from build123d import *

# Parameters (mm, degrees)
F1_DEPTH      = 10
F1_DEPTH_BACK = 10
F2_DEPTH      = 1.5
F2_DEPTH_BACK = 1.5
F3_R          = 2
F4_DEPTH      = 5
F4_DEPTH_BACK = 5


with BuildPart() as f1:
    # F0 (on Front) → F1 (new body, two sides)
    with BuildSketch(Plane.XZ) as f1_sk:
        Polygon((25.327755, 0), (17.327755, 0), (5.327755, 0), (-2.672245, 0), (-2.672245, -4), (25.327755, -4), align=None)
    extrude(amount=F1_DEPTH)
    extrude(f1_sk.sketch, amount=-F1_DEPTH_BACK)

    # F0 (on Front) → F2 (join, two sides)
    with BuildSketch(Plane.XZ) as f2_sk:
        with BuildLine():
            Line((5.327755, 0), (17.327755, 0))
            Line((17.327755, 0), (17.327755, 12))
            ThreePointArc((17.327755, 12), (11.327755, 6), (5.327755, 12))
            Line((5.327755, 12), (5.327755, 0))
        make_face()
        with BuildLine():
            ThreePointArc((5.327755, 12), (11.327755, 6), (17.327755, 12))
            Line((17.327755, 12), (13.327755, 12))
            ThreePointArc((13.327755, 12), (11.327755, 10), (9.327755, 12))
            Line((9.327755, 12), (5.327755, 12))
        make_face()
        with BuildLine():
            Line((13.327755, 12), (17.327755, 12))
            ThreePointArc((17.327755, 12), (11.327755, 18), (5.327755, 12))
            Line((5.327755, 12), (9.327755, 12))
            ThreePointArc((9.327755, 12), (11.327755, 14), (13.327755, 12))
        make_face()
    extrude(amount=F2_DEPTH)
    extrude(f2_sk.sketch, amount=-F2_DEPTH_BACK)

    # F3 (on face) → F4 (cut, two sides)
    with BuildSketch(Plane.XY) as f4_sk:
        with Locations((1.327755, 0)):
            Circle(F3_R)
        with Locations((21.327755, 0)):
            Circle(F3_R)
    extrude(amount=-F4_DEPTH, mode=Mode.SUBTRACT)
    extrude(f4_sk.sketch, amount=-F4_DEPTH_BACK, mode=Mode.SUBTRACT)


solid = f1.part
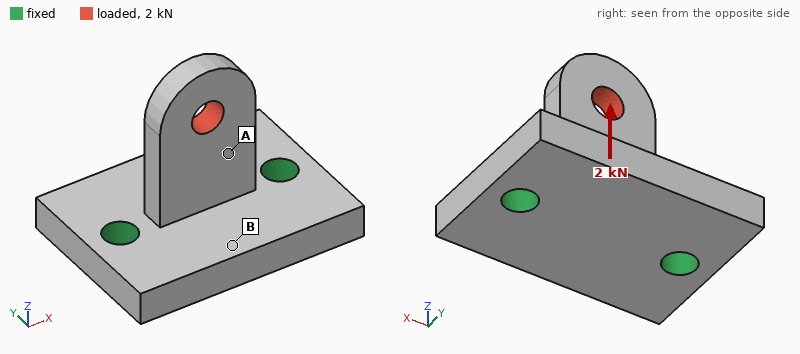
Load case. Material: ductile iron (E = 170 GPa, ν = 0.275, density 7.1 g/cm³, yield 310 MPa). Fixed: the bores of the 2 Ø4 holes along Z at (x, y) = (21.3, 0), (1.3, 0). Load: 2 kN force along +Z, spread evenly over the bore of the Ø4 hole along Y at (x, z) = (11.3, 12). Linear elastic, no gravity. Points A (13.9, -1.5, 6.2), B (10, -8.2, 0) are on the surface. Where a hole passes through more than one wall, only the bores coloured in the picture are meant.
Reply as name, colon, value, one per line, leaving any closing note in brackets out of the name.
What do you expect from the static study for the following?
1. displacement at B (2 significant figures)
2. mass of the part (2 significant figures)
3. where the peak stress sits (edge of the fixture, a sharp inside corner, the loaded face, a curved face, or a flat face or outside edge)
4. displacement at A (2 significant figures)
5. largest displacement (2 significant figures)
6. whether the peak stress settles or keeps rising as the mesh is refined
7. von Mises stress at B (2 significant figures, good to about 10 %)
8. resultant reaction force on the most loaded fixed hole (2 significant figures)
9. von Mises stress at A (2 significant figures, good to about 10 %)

displacement at B: 3.1 µm
mass of the part: 19 g
where the peak stress sits: edge of the fixture
displacement at A: 5.7 µm
largest displacement: 10.0 µm
whether the peak stress settles or keeps rising as the mesh is refined: keeps rising
von Mises stress at B: 22 MPa
resultant reaction force on the most loaded fixed hole: 1.0 kN
von Mises stress at A: 57 MPa
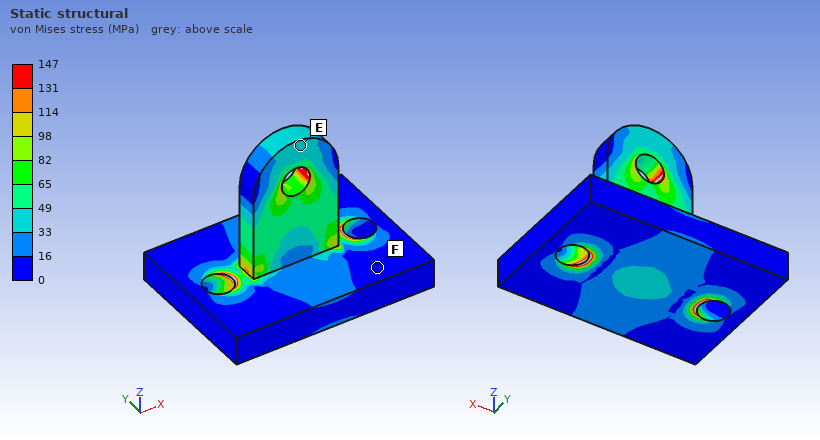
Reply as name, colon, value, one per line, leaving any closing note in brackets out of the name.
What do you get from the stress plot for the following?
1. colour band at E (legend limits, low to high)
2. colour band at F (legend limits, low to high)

colour band at E: 33 to 49 MPa
colour band at F: 0 to 16 MPa
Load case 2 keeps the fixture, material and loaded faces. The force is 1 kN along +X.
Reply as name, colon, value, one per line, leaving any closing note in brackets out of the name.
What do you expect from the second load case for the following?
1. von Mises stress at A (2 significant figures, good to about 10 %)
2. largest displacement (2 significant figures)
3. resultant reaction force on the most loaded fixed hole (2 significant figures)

von Mises stress at A: 64 MPa
largest displacement: 31 µm
resultant reaction force on the most loaded fixed hole: 1.0 kN
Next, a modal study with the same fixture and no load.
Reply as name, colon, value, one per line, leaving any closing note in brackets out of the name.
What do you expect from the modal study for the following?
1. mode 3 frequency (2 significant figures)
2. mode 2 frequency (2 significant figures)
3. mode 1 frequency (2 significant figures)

mode 3 frequency: 24 kHz
mode 2 frequency: 21 kHz
mode 1 frequency: 7300 Hz
